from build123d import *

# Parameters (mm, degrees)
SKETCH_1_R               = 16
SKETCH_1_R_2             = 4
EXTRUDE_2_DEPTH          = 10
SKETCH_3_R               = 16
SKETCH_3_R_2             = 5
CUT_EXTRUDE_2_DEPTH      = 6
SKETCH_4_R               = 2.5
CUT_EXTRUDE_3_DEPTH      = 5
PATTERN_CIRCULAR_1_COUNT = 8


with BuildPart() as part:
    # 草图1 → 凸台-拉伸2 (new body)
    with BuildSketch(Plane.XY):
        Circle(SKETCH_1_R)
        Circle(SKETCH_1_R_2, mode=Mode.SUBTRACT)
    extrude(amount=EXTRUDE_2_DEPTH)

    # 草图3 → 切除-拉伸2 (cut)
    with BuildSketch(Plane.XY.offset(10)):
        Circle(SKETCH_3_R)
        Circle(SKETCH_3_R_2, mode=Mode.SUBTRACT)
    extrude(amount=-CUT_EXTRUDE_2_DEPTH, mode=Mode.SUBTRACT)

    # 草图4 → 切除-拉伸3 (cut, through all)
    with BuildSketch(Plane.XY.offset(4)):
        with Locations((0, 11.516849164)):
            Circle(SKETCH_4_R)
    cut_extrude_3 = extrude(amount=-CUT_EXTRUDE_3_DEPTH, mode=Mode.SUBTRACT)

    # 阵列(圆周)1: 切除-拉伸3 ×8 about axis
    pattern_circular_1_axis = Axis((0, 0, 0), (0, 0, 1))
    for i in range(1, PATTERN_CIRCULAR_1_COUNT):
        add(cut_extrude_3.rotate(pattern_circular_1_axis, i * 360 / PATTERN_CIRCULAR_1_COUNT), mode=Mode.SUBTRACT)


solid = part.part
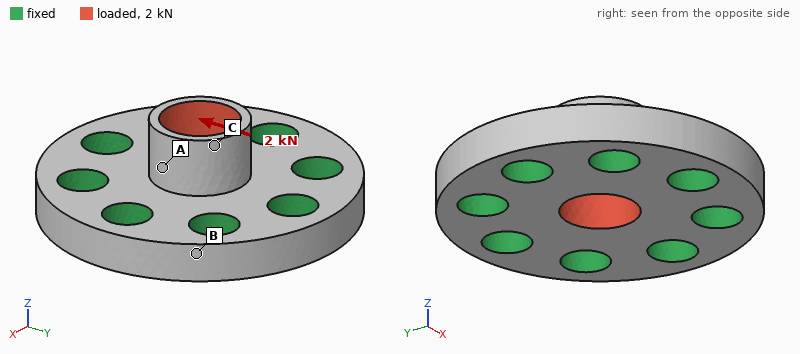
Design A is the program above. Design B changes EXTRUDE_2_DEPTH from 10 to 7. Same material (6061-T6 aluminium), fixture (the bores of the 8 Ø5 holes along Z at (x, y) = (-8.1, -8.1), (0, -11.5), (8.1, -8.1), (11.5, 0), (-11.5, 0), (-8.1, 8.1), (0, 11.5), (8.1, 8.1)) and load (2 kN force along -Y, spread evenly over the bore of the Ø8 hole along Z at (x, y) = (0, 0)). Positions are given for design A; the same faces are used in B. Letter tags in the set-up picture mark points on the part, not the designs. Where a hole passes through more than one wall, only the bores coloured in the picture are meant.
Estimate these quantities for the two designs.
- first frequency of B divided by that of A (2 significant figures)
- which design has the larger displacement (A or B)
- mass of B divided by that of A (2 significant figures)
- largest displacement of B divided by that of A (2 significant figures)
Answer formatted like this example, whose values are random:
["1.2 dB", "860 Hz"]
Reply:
["1.6", "A", "0.97", "0.50"]
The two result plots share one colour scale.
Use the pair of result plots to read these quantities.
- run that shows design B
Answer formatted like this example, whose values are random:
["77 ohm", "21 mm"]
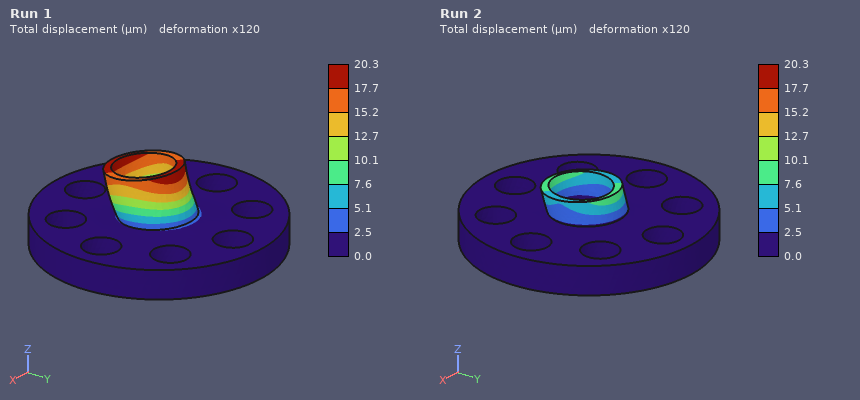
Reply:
["Run 2"]
